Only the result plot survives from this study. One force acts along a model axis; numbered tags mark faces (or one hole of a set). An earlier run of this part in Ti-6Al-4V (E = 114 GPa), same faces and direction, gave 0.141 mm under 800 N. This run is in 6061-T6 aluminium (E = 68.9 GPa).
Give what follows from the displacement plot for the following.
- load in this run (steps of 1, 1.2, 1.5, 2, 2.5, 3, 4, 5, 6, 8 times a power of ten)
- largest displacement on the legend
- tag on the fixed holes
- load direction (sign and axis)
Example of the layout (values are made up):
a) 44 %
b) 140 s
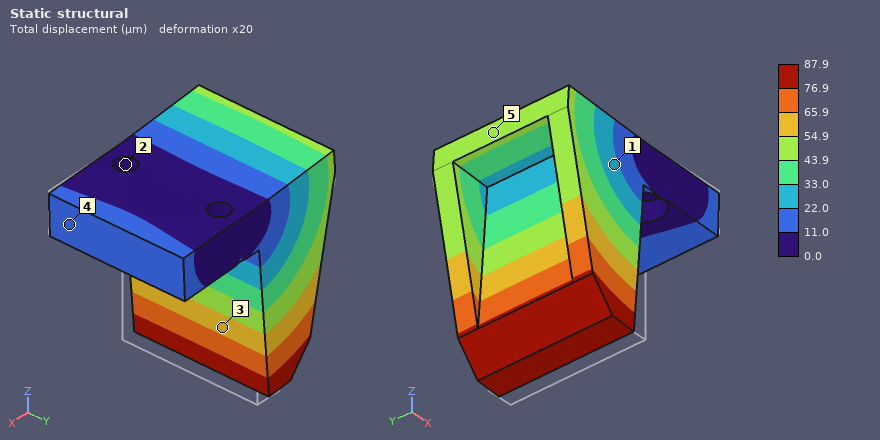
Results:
a) 300 N
b) 87.9 µm
c) 2
d) -X
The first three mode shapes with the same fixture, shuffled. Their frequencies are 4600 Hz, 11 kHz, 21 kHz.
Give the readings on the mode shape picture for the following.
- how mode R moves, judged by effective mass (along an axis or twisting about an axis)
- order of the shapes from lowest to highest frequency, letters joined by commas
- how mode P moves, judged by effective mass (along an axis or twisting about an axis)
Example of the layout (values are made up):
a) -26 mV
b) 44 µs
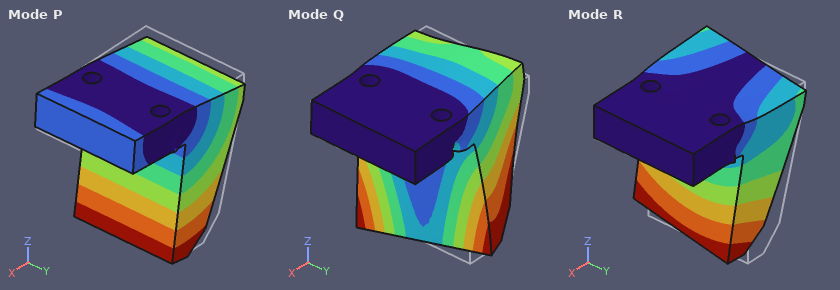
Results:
a) along Y
b) P, R, Q
c) along X
